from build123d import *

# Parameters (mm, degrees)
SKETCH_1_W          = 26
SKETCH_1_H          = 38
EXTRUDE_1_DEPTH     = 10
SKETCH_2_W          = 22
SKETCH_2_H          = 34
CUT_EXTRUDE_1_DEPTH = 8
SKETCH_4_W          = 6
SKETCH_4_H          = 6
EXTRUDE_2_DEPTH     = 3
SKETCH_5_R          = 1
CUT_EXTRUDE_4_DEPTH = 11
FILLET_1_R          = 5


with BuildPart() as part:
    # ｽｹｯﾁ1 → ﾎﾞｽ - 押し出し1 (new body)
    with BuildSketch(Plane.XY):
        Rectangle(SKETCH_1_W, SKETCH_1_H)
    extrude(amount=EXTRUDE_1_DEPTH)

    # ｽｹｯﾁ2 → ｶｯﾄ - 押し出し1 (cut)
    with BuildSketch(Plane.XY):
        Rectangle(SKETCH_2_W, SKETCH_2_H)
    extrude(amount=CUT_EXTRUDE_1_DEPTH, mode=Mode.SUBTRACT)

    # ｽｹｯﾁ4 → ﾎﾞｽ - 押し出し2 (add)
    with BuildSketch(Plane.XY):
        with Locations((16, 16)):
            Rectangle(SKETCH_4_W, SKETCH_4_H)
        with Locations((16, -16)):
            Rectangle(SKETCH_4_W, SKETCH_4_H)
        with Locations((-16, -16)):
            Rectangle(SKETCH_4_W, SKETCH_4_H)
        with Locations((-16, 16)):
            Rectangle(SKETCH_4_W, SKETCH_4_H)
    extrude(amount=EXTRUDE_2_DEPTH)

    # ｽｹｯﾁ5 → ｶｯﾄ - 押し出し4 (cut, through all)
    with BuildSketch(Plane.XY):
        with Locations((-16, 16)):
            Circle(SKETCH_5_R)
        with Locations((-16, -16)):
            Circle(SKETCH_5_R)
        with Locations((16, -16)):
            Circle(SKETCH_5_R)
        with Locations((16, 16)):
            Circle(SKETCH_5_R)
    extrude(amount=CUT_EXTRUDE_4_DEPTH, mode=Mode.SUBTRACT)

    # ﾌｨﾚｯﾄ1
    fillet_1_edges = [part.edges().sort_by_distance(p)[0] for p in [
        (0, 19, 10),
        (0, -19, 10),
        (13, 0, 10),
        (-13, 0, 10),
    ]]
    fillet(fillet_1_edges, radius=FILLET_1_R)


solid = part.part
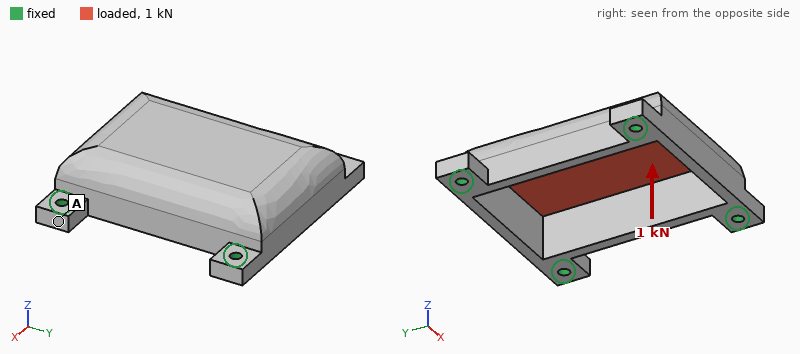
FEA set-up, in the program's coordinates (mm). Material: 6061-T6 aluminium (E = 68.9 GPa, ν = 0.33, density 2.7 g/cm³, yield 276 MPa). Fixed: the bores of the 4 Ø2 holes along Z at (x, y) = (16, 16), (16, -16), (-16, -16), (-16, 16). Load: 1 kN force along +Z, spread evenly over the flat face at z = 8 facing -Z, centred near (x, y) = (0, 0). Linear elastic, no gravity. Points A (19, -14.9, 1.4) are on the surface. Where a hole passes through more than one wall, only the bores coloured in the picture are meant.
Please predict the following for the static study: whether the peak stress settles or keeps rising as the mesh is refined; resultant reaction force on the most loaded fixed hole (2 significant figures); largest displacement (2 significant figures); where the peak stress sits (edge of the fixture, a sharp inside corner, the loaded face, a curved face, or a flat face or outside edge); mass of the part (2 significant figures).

keeps rising
300 N
53 µm
edge of the fixture
9.9 g
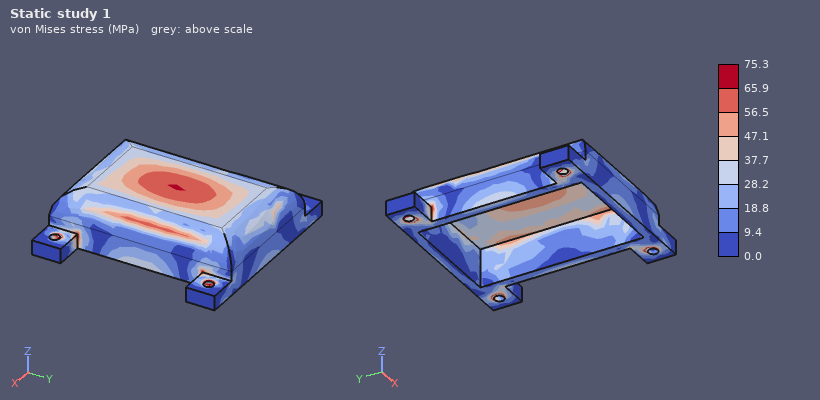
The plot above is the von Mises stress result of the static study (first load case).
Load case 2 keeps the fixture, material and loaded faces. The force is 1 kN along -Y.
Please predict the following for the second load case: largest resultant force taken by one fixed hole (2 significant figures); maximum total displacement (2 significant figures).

270 N
11 µm
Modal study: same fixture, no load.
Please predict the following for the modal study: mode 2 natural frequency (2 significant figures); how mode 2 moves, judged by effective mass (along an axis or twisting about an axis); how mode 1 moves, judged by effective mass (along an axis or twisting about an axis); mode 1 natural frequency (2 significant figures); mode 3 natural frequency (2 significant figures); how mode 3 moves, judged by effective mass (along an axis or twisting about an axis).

17 kHz
along X
along Z
13 kHz
18 kHz
along Y
